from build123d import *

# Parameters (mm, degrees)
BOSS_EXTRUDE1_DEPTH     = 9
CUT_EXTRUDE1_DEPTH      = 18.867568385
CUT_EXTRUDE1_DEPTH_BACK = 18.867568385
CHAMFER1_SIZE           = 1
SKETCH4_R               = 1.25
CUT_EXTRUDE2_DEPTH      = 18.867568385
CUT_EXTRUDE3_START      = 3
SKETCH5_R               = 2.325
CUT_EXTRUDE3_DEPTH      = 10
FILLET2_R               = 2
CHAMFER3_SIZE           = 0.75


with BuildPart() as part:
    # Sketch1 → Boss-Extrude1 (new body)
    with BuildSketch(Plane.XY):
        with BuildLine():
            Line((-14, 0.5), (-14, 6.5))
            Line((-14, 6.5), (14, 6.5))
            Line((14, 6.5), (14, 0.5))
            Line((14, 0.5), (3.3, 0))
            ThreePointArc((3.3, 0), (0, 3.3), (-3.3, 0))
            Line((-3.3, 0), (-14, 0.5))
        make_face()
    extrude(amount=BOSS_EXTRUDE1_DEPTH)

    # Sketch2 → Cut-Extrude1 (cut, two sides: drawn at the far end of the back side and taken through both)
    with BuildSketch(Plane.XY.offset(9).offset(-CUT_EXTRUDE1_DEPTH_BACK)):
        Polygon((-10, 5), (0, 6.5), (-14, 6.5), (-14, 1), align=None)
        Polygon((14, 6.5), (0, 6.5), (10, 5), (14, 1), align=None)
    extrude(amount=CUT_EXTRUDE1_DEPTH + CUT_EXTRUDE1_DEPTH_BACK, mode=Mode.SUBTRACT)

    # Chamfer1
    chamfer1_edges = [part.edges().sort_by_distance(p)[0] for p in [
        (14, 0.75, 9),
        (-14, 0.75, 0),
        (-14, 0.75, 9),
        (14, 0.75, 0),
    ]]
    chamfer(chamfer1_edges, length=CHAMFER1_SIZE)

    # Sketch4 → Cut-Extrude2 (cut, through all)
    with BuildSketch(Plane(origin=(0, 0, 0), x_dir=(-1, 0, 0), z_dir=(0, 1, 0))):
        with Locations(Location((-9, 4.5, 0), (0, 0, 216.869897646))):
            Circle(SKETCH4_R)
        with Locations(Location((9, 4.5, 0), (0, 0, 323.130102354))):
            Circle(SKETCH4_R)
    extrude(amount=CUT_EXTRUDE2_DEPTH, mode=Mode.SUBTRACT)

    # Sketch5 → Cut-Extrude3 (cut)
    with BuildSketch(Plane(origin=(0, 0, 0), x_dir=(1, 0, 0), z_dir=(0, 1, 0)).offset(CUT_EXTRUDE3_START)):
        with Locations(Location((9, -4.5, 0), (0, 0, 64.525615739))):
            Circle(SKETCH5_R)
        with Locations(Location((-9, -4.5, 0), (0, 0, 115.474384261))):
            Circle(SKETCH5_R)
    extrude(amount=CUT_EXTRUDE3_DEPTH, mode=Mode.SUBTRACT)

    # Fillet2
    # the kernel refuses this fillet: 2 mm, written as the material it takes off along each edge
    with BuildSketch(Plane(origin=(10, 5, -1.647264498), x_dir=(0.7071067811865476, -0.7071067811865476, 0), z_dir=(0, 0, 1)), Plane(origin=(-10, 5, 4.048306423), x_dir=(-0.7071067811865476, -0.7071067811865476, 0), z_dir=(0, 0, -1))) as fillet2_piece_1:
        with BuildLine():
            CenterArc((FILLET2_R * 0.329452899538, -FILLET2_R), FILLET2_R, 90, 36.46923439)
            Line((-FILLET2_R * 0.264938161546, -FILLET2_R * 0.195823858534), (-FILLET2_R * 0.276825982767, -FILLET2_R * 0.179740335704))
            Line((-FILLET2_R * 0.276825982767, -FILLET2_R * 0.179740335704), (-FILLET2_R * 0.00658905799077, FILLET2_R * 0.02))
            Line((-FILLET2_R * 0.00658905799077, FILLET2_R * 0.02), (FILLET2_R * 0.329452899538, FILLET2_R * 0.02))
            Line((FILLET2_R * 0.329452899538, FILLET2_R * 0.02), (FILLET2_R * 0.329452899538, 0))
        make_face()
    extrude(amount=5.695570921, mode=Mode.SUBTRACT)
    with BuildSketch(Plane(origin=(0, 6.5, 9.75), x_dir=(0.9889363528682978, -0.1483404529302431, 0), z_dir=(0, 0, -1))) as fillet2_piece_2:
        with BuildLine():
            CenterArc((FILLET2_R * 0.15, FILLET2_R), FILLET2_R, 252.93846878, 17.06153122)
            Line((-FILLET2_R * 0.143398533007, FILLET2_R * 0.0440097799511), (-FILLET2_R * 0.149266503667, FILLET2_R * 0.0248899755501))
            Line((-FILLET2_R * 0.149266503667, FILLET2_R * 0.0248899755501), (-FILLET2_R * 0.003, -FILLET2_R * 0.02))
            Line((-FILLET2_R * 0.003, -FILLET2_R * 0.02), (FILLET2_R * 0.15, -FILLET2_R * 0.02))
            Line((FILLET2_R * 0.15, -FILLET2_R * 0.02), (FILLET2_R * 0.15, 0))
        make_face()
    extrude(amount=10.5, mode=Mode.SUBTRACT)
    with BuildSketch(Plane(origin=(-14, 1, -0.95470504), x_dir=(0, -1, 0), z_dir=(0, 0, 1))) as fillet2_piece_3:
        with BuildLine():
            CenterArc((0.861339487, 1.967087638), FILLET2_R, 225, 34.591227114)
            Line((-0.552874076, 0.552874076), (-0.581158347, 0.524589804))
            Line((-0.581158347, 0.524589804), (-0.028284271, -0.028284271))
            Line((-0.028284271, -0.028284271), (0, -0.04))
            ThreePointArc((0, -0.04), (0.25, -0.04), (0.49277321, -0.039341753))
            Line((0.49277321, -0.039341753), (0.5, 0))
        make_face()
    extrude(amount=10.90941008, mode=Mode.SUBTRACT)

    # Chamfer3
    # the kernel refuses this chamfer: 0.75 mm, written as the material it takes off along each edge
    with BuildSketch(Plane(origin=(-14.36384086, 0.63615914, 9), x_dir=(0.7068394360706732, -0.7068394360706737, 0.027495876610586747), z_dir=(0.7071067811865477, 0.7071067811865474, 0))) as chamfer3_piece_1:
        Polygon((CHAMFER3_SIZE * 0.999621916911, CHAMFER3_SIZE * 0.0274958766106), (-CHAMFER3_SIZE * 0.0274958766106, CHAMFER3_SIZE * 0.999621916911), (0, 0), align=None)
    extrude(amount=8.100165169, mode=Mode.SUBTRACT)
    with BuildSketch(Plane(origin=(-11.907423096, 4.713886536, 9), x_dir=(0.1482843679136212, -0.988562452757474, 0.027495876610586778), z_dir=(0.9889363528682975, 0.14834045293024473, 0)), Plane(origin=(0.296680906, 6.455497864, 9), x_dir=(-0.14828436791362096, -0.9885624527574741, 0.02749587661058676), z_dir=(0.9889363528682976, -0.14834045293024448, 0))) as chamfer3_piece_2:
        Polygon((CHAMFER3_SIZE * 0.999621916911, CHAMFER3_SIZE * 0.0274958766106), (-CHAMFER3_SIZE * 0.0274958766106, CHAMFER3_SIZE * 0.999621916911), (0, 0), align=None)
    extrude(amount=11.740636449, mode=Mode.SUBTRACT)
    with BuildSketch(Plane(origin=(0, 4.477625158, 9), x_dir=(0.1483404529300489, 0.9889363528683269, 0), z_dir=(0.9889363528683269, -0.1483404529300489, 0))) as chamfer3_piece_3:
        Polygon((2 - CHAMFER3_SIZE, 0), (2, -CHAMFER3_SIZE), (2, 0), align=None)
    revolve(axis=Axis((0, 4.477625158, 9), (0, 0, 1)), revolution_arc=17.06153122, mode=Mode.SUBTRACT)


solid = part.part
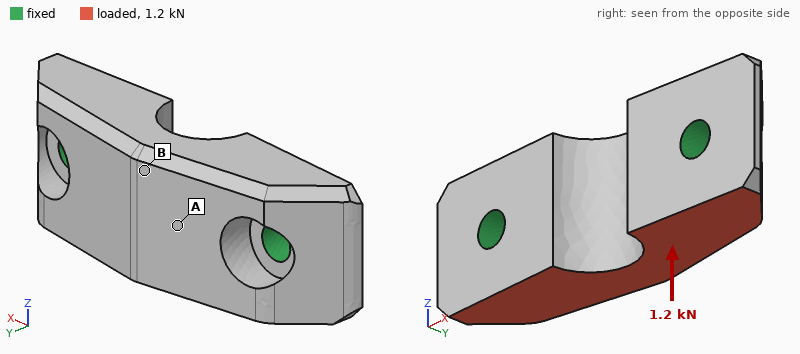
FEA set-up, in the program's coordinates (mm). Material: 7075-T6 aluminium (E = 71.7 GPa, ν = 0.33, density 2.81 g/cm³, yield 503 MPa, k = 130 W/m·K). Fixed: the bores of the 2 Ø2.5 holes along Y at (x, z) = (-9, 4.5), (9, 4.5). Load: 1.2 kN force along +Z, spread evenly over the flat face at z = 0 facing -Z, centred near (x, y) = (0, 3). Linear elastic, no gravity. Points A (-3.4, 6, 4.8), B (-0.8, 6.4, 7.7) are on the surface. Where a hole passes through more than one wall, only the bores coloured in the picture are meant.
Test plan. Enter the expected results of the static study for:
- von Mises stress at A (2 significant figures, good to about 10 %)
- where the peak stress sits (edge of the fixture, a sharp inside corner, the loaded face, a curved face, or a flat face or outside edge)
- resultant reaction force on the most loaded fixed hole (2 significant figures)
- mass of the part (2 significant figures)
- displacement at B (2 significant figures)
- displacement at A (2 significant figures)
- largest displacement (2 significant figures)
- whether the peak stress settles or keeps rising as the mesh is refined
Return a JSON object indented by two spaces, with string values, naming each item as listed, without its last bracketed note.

{
  "von Mises stress at A": "24 MPa",
  "where the peak stress sits": "edge of the fixture",
  "resultant reaction force on the most loaded fixed hole": "600 N",
  "mass of the part": "2.7 g",
  "displacement at B": "10 µm",
  "displacement at A": "8.5 µm",
  "largest displacement": "12 µm",
  "whether the peak stress settles or keeps rising as the mesh is refined": "keeps rising"
}
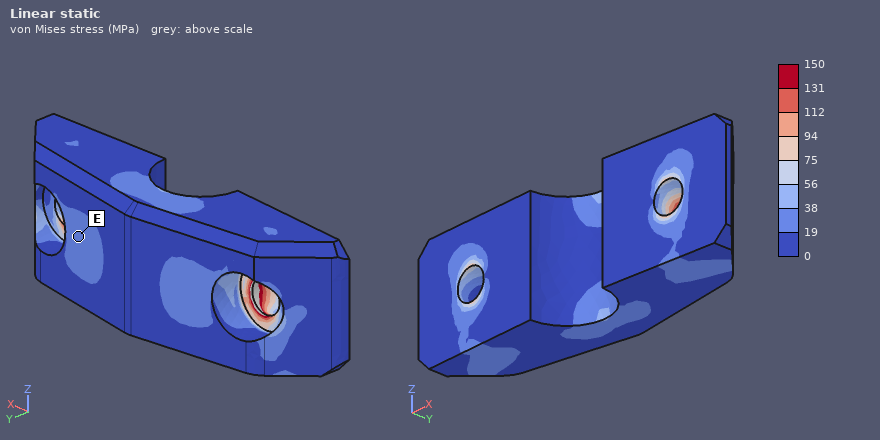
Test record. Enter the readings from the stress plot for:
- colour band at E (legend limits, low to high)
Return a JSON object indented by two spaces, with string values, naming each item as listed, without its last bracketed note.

{
  "colour band at E": "19 to 38 MPa"
}
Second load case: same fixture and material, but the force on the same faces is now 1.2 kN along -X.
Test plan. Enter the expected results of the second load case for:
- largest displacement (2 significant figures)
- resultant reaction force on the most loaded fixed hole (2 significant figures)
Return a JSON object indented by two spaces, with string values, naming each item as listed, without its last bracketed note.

{
  "largest displacement": "5.4 µm",
  "resultant reaction force on the most loaded fixed hole": "650 N"
}
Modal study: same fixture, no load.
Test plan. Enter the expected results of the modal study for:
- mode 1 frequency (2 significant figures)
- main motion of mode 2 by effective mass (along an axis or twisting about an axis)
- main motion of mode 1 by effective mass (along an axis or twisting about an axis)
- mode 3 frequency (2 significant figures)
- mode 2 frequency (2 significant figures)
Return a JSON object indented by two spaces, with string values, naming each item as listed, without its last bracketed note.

{
  "mode 1 frequency": "36 kHz",
  "main motion of mode 2 by effective mass": "along Y",
  "main motion of mode 1 by effective mass": "along Z",
  "mode 3 frequency": "65 kHz",
  "mode 2 frequency": "51 kHz"
}
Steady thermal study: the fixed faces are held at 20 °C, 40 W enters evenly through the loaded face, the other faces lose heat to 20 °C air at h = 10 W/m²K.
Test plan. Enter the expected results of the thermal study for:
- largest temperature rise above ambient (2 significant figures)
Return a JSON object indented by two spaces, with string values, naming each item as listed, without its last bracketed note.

{
  "largest temperature rise above ambient": "26 K"
}
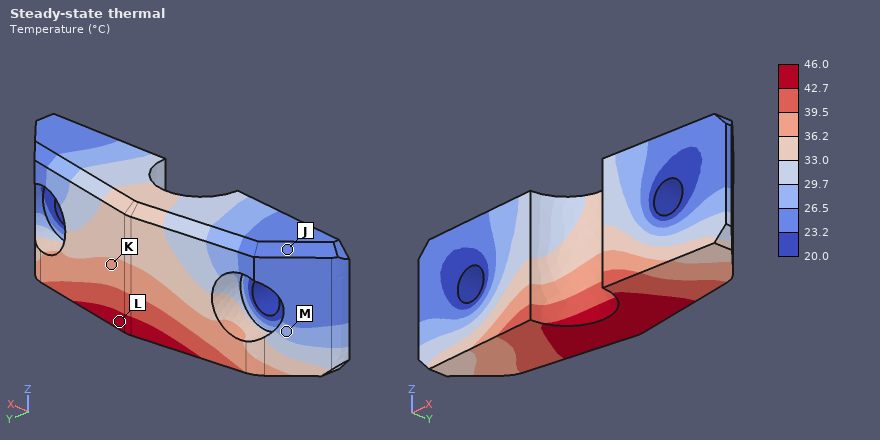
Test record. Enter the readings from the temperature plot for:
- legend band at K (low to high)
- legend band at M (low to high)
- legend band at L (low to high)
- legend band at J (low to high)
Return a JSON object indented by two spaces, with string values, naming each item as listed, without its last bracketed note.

{
  "legend band at K": "36.2 to 39.5 °C",
  "legend band at M": "26.5 to 29.7 °C",
  "legend band at L": "42.7 to 46.0 °C",
  "legend band at J": "23.2 to 26.5 °C"
}
